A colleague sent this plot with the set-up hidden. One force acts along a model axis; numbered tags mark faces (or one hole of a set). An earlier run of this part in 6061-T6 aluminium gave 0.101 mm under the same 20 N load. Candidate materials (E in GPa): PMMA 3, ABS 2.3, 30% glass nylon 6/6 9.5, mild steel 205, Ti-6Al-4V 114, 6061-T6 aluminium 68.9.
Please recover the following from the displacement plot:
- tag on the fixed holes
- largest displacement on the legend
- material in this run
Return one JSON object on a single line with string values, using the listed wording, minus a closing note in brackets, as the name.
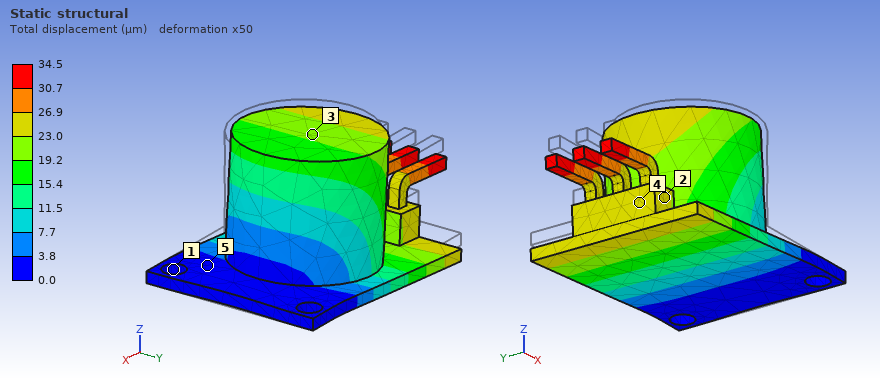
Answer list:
{"tag on the fixed holes": "1", "largest displacement on the legend": "34.5 µm", "material in this run": "mild steel"}
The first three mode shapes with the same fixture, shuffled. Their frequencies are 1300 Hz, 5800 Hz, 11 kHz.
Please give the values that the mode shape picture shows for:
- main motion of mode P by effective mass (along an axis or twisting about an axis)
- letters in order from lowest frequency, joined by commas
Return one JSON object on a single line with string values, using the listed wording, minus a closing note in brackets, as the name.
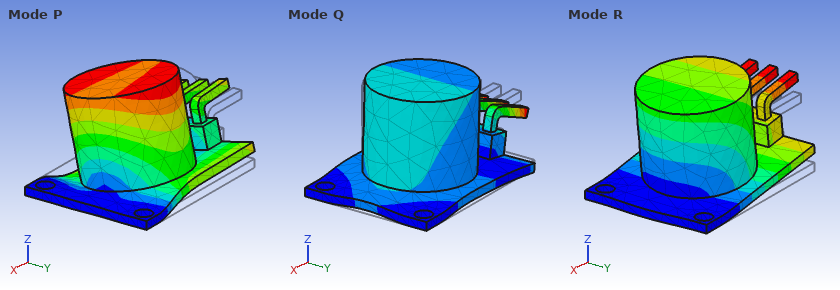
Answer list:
{"main motion of mode P by effective mass": "along Y", "letters in order from lowest frequency, joined by commas": "R, P, Q"}
